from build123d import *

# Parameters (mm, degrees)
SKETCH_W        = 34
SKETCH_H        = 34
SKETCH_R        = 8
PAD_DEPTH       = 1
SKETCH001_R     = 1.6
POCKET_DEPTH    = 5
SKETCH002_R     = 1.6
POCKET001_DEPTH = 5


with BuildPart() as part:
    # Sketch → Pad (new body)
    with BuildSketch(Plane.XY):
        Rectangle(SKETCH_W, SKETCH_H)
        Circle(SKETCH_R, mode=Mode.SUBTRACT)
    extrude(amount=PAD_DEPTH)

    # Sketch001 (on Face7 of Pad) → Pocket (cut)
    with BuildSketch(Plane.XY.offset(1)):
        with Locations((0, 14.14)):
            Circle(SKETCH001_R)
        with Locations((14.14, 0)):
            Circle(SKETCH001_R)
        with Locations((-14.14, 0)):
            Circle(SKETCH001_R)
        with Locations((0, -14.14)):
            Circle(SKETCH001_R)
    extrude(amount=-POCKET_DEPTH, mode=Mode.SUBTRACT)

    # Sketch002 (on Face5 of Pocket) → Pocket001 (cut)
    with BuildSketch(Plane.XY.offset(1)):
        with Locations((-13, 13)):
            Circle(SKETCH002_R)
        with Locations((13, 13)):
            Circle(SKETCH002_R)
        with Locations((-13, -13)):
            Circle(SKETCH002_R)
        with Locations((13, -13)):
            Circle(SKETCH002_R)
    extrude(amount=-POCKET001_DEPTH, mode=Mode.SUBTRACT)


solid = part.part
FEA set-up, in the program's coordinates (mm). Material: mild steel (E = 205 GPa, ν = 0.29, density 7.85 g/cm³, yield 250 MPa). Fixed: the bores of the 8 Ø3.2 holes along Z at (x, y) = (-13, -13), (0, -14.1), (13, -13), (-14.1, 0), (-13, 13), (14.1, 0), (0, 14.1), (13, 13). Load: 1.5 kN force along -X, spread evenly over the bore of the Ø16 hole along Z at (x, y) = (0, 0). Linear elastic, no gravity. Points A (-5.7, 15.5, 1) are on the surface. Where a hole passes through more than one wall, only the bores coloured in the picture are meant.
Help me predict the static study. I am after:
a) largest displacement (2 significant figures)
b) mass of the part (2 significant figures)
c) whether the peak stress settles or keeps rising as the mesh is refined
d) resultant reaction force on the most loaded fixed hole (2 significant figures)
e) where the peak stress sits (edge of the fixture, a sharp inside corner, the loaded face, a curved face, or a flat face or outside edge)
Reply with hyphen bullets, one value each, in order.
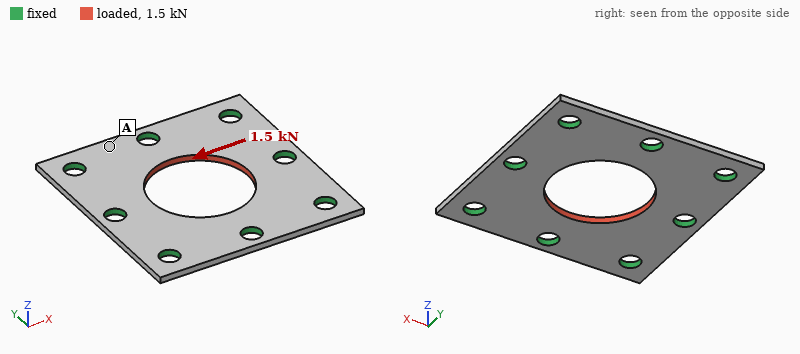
- 1.5 µm
- 7.0 g
- keeps rising
- 320 N
- edge of the fixture
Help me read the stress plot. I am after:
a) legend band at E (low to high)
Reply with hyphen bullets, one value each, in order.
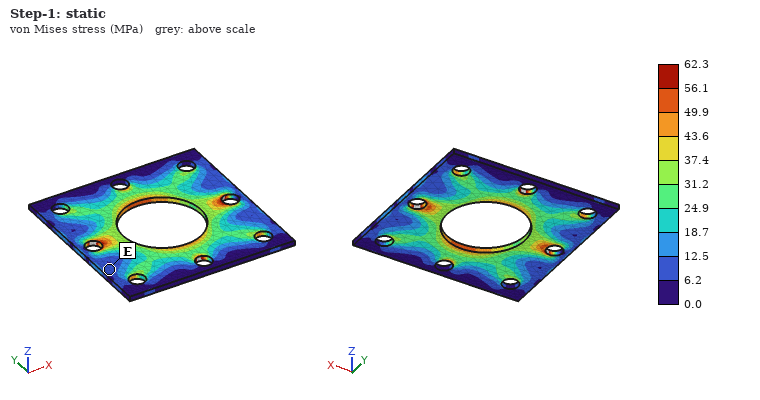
- 6.2 to 12.5 MPa
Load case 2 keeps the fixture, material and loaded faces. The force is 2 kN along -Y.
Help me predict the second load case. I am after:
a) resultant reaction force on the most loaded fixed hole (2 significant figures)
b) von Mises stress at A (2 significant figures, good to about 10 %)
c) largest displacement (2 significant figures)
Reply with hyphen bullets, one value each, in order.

- 420 N
- 9.6 MPa
- 2.0 µm
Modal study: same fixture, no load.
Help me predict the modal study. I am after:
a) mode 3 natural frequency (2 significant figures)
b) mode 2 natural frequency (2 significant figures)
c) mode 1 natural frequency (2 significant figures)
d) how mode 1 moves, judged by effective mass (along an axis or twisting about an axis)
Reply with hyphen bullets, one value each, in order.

- 24 kHz
- 24 kHz
- 22 kHz
- along Z
